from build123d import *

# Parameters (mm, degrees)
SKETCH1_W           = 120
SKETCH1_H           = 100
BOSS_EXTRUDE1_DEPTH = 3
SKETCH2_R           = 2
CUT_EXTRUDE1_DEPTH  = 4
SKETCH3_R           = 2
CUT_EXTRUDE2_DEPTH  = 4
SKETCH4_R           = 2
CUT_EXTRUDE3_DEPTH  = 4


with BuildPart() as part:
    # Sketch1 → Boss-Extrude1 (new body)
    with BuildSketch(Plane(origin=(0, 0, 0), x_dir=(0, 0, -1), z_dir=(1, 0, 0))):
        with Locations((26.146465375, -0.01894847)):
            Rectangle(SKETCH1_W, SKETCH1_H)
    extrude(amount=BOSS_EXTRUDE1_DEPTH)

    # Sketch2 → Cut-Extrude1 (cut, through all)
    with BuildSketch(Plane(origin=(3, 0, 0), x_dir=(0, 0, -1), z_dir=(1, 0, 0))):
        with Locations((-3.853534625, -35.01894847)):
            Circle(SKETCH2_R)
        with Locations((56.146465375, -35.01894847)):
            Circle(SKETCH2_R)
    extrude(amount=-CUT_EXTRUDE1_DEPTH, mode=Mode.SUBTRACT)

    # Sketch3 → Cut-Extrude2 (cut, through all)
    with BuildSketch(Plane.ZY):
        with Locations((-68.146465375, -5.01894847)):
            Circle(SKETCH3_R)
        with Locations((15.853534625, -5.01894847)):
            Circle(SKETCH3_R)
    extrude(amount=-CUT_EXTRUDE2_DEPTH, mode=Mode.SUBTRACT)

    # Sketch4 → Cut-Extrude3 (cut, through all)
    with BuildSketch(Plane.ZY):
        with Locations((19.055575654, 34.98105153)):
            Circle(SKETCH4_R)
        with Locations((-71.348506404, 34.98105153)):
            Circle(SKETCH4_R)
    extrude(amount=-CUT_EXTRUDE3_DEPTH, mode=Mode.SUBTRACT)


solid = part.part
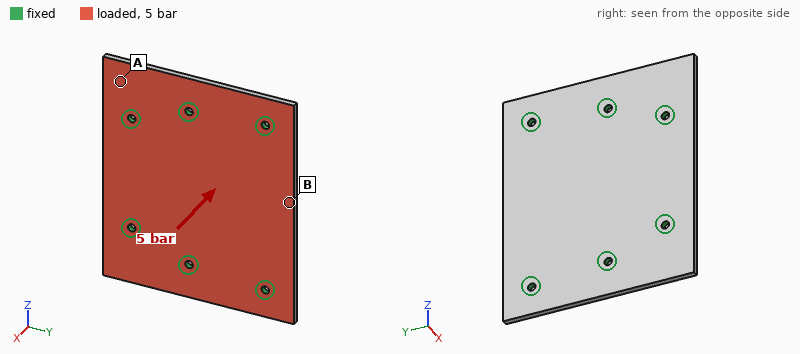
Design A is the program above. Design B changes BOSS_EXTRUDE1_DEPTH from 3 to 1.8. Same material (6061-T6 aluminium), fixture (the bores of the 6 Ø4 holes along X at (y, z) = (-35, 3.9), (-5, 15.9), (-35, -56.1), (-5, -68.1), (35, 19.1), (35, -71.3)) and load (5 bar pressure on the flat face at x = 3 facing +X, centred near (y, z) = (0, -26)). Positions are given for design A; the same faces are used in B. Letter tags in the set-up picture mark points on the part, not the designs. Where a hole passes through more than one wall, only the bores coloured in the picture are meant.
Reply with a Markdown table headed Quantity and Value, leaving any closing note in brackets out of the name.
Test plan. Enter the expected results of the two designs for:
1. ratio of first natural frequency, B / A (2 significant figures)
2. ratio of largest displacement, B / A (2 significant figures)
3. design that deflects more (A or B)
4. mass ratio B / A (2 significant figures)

| Quantity | Value |
|---|---|
| ratio of first natural frequency, B / A | 0.62 |
| ratio of largest displacement, B / A | 4.4 |
| design that deflects more | B |
| mass ratio B / A | 0.60 |
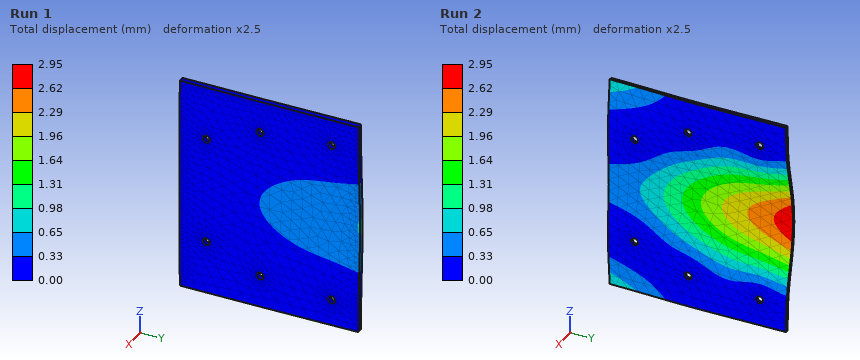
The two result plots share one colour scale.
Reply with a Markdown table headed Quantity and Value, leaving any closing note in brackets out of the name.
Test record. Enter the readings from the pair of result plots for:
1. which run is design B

| Quantity | Value |
|---|---|
| which run is design B | Run 2 |
